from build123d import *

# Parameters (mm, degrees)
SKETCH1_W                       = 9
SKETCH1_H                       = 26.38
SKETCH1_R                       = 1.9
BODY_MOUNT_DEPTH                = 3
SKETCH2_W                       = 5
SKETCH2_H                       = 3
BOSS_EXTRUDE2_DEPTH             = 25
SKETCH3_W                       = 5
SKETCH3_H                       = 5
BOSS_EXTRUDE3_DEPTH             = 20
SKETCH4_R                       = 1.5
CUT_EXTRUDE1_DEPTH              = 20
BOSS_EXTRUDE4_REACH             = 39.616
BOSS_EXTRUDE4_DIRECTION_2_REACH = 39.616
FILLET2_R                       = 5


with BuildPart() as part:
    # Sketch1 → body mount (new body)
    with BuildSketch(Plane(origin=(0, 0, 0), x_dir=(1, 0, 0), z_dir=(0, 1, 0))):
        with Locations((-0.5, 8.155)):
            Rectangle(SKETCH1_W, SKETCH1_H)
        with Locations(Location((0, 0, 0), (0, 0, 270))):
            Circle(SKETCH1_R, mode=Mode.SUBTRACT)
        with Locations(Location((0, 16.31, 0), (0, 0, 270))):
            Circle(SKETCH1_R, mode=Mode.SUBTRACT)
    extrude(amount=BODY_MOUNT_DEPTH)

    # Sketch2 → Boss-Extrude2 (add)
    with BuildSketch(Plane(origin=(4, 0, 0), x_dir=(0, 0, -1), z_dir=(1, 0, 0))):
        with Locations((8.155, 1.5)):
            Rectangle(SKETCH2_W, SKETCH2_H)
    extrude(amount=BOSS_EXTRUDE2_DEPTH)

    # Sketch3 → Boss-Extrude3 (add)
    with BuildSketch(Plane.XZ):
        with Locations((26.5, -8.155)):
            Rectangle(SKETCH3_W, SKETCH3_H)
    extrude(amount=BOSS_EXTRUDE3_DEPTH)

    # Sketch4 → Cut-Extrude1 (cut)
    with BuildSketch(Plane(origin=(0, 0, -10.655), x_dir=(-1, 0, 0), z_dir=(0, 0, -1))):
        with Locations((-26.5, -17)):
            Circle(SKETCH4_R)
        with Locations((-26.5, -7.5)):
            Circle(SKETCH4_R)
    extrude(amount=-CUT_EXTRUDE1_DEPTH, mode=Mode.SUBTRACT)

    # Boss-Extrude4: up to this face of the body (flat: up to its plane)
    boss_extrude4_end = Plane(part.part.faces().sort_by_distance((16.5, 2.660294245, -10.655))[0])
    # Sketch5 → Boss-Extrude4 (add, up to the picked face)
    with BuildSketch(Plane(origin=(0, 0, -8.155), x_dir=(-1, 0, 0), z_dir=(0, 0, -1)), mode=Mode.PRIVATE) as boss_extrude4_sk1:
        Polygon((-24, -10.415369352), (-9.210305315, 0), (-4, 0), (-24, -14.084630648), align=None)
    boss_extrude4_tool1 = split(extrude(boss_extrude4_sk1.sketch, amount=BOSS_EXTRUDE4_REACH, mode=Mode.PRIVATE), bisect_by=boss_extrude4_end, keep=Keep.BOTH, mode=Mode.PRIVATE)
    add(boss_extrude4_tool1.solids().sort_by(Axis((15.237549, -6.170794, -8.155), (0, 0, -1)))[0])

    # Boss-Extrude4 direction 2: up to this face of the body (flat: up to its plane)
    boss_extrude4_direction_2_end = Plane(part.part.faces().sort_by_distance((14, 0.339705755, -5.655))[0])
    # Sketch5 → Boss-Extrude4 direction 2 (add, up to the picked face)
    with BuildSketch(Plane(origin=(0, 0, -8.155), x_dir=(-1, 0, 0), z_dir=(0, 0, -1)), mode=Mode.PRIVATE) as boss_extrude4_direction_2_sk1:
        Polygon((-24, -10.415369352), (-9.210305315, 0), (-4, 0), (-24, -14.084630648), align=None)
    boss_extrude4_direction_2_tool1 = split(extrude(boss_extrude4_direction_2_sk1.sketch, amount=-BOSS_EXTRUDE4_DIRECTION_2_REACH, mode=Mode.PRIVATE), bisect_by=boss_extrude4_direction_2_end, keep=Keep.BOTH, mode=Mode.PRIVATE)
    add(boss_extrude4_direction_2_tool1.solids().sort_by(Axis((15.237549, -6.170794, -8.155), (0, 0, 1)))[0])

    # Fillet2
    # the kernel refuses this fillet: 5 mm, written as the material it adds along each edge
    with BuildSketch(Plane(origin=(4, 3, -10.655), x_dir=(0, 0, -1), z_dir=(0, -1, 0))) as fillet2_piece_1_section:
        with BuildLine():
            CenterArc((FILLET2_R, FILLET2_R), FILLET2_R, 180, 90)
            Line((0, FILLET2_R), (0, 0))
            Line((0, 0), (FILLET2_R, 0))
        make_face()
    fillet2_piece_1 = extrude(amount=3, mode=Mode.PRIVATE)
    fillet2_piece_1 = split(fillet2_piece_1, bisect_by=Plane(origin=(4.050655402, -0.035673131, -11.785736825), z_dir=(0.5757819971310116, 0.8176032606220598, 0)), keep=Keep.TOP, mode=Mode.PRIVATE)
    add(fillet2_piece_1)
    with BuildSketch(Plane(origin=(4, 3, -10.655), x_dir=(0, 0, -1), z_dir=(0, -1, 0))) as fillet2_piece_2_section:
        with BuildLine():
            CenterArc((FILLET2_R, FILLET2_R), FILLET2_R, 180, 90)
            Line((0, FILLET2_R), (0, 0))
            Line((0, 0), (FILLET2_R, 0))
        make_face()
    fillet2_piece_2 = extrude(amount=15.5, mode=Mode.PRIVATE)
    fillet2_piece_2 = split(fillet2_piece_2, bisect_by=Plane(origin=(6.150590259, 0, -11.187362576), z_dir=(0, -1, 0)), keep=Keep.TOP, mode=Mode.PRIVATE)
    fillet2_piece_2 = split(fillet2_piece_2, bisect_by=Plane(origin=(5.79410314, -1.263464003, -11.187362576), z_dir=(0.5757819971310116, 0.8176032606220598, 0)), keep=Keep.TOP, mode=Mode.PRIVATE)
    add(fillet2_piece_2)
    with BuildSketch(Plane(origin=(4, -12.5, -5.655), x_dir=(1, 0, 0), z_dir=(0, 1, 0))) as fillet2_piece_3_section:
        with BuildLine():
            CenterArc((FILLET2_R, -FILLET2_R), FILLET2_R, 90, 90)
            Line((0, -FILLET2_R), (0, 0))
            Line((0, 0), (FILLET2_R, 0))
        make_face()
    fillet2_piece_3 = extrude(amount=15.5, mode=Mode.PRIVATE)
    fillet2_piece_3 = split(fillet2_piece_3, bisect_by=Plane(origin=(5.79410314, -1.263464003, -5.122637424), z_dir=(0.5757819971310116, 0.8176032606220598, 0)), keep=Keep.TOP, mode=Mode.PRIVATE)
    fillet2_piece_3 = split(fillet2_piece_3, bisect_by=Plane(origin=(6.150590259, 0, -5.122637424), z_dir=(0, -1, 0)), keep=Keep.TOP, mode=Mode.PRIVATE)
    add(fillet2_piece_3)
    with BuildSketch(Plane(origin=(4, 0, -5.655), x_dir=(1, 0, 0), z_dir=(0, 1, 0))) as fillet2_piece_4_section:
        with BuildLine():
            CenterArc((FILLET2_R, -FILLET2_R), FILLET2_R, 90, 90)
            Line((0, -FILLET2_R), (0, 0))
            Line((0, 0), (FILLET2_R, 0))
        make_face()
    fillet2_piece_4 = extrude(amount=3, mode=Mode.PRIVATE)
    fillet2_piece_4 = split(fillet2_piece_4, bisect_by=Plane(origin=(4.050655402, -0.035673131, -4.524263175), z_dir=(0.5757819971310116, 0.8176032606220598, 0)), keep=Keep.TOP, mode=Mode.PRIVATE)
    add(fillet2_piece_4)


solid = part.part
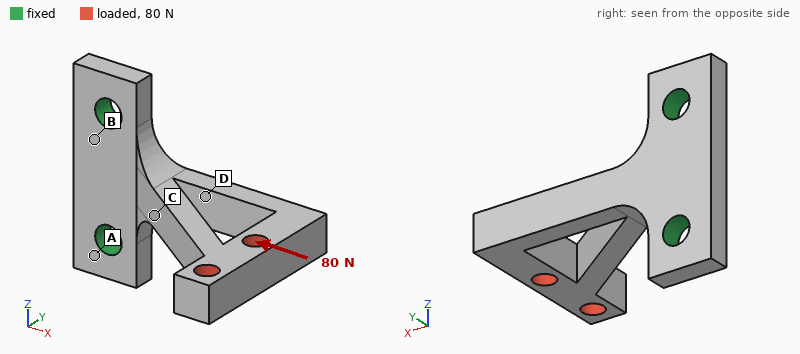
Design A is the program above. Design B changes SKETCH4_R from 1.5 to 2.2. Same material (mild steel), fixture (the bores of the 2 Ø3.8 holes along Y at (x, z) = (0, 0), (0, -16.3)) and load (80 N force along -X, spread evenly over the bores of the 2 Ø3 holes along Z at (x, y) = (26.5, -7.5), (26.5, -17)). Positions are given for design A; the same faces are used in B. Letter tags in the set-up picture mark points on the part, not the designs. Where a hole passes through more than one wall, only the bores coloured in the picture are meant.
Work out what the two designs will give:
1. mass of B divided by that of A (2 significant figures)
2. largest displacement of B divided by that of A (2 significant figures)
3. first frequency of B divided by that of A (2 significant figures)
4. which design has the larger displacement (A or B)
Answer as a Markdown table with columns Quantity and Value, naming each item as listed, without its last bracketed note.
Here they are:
| Quantity | Value |
|---|---|
| mass of B divided by that of A | 0.96 |
| largest displacement of B divided by that of A | 1.1 |
| first frequency of B divided by that of A | 1.1 |
| which design has the larger displacement | B |
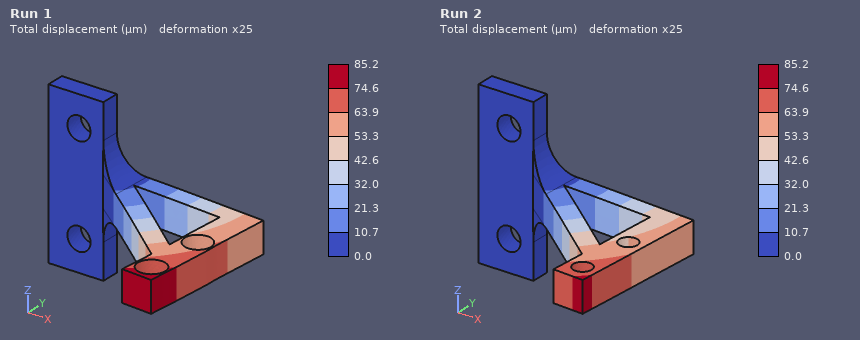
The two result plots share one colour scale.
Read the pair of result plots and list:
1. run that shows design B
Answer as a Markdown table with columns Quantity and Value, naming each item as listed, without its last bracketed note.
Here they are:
| Quantity | Value |
|---|---|
| run that shows design B | Run 1 |
